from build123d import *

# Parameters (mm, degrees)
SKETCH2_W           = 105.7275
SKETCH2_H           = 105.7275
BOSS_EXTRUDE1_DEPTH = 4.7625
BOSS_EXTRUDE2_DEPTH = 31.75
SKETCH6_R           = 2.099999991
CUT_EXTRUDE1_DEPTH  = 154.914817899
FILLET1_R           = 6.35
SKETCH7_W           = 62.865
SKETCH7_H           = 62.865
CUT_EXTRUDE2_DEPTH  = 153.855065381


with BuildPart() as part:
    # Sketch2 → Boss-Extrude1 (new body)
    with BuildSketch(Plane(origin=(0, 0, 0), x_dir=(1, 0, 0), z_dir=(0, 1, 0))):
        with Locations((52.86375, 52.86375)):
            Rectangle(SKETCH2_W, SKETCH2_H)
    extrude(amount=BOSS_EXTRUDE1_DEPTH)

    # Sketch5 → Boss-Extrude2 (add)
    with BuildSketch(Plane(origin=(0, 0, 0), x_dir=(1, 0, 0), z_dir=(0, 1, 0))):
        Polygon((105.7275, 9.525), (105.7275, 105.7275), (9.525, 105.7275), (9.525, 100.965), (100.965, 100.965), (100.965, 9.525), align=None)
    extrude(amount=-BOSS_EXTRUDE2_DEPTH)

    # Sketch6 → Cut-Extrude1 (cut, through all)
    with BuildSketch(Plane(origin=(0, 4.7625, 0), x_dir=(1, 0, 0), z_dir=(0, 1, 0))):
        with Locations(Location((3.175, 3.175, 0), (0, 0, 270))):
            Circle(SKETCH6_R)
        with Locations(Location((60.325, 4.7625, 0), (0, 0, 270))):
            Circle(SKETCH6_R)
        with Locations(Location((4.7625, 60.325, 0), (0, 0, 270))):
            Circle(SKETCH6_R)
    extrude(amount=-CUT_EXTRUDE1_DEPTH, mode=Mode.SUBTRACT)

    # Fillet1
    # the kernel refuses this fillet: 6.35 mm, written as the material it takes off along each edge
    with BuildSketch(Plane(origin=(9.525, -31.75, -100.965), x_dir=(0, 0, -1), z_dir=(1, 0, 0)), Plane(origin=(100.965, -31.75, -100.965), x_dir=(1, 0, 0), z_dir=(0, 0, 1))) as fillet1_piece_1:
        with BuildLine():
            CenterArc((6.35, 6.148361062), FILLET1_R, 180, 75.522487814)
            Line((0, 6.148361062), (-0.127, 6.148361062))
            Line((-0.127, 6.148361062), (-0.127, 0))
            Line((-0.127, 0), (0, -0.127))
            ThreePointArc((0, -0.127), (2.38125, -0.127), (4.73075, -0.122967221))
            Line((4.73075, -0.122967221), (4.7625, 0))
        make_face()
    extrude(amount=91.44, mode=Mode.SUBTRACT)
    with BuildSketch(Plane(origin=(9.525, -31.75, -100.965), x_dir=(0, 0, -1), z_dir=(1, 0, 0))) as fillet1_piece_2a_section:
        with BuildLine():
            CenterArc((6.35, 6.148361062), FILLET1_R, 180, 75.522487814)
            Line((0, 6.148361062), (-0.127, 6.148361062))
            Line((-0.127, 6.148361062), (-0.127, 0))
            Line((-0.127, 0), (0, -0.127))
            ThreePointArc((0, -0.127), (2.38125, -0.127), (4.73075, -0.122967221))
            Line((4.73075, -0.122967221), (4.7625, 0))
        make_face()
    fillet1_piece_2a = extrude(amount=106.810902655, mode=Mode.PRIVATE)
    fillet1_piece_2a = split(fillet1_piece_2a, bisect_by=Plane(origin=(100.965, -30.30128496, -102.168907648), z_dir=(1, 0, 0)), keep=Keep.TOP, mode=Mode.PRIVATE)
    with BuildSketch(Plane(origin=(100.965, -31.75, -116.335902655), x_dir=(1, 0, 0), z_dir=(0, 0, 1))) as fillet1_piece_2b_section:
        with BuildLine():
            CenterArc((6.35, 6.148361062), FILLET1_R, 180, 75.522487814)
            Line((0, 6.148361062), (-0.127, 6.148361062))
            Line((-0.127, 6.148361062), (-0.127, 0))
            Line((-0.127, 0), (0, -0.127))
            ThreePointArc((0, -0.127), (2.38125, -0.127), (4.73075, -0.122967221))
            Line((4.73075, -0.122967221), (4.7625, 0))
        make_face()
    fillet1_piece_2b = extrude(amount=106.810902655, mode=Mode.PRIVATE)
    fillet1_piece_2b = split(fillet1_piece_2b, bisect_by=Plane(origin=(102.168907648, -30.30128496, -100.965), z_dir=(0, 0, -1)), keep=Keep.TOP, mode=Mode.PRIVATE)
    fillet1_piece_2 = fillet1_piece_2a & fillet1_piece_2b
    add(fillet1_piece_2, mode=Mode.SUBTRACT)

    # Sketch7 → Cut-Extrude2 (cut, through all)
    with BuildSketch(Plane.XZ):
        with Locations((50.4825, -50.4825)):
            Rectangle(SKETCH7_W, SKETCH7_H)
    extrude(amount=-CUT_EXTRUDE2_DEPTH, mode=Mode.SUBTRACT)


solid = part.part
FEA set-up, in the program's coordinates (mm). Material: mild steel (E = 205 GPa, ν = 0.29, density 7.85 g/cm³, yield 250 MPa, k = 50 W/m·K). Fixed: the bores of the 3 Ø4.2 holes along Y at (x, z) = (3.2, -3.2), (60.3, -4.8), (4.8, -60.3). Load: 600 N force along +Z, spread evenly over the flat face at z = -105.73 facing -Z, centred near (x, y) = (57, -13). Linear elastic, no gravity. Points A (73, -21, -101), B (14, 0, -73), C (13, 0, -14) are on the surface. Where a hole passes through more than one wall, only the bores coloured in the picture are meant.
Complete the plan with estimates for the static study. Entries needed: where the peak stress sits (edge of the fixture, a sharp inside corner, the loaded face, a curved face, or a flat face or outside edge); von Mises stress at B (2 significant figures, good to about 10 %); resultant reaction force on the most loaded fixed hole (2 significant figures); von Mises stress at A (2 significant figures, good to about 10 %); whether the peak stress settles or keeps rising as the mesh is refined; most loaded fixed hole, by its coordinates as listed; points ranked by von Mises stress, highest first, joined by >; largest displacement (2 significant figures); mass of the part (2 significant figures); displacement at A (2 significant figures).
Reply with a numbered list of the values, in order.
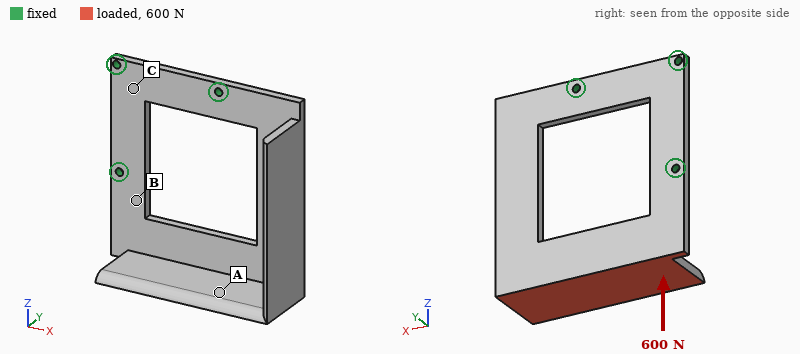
1. edge of the fixture
2. 61 MPa
3. 450 N
4. 15 MPa
5. keeps rising
6. (60.3, -4.8)
7. B > A > C
8. 0.32 mm
9. 480 g
10. 0.23 mm
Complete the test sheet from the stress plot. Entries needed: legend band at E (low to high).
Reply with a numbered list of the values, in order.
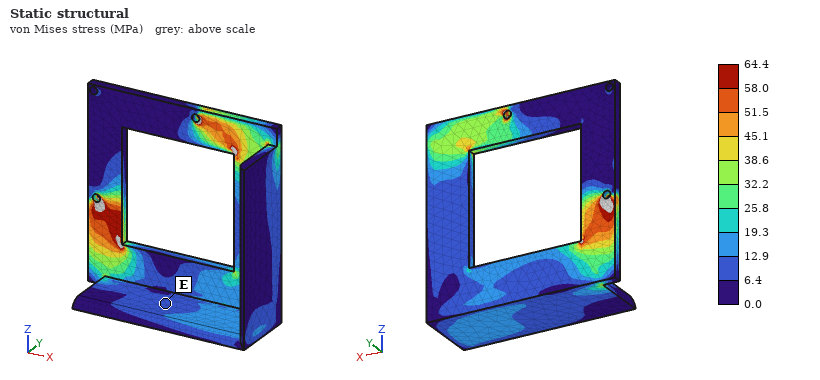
1. 6.4 to 12.9 MPa
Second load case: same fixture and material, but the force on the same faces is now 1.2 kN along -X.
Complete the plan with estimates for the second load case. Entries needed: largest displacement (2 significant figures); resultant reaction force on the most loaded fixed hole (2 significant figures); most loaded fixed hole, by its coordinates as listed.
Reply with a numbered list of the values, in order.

1. 0.70 mm
2. 1.7 kN
3. (4.8, -60.3)
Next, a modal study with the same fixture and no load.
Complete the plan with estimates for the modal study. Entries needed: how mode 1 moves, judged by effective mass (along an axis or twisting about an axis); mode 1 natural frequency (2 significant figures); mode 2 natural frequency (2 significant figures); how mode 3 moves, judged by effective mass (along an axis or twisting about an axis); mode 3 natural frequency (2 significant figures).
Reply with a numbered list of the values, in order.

1. along Y
2. 220 Hz
3. 810 Hz
4. along Y
5. 1400 Hz
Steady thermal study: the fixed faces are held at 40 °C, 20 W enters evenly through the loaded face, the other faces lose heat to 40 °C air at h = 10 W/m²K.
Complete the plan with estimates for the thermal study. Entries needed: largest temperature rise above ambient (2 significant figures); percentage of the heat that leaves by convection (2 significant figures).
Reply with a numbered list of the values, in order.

1. 77 K
2. 50 %
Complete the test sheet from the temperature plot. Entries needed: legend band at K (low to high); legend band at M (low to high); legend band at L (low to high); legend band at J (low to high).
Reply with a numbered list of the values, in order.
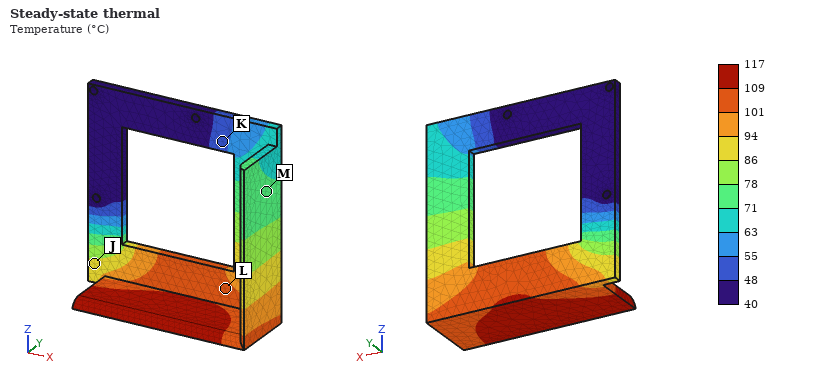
1. 48 to 55 °C
2. 71 to 78 °C
3. 101 to 109 °C
4. 86 to 94 °C
